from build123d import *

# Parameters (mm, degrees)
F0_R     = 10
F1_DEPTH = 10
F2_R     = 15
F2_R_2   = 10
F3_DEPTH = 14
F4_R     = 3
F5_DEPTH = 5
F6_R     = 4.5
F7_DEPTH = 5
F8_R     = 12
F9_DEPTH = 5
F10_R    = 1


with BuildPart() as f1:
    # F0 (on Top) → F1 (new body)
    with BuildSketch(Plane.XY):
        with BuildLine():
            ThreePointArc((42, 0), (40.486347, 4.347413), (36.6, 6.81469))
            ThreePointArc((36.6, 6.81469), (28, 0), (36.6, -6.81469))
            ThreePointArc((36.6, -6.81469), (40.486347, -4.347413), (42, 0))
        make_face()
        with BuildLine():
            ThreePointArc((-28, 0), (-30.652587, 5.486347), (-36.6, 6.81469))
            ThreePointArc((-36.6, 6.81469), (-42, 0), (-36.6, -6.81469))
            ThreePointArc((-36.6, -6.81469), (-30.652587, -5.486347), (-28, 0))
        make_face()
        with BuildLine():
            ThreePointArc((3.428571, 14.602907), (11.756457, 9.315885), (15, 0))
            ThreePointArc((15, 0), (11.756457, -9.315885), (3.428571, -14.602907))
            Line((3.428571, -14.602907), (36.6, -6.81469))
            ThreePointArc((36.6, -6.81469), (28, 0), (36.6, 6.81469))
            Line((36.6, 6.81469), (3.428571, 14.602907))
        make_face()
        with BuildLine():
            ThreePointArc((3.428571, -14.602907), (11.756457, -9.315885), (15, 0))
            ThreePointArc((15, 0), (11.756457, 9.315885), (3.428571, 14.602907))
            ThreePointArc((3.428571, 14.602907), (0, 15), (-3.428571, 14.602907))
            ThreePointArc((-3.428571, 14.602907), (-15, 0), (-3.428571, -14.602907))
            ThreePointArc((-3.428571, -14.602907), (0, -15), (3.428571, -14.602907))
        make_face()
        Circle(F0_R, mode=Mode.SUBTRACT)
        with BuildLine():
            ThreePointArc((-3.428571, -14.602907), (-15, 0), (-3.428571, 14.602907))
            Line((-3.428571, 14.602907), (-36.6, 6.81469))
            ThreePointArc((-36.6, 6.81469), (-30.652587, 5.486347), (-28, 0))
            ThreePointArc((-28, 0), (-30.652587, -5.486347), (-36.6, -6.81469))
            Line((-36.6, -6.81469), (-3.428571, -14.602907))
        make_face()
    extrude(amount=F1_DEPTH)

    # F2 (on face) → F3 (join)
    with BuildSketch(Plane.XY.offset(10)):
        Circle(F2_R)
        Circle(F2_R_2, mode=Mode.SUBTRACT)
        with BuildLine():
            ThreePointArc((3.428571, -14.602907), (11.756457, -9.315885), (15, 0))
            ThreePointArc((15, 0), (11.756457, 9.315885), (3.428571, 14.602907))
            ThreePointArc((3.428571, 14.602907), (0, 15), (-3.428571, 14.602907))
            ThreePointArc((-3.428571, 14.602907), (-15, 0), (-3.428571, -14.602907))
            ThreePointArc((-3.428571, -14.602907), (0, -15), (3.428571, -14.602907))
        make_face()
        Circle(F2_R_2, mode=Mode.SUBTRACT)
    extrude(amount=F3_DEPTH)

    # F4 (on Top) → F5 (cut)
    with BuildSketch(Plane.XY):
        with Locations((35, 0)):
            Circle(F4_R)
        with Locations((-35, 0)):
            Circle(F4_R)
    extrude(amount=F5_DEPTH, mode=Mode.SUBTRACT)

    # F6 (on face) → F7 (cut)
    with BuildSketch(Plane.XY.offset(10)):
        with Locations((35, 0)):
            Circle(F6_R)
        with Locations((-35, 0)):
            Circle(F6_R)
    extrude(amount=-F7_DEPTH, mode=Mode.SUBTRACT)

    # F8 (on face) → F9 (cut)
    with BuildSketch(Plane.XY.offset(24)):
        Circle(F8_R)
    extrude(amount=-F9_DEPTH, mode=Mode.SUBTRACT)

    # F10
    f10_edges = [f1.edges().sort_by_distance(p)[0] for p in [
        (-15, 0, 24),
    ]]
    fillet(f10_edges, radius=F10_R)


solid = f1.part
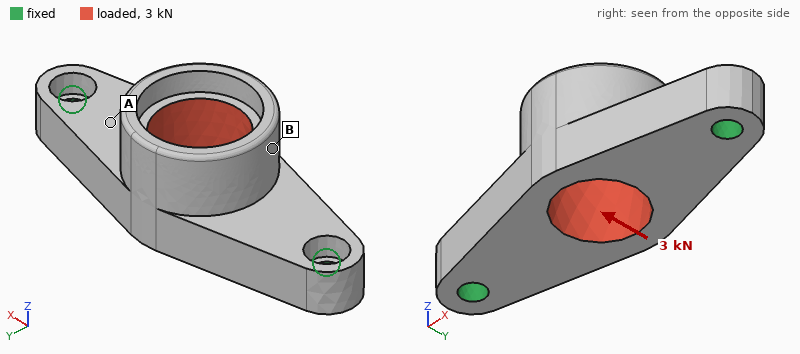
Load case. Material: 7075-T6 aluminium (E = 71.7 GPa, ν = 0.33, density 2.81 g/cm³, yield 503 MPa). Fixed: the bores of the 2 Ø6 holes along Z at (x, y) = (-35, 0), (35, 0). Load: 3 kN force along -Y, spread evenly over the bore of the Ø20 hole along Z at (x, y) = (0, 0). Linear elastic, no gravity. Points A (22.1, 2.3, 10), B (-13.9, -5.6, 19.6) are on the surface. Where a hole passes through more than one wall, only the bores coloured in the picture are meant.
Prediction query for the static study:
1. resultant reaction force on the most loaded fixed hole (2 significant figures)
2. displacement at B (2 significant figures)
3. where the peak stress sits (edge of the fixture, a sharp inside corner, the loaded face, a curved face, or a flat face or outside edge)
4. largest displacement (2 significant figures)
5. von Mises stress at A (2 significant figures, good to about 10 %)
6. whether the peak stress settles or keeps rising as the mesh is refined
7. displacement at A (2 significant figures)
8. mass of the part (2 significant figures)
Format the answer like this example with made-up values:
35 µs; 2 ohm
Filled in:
1.5 kN; 62 µm; edge of the fixture; 82 µm; 41 MPa; keeps rising; 26 µm; 51 g
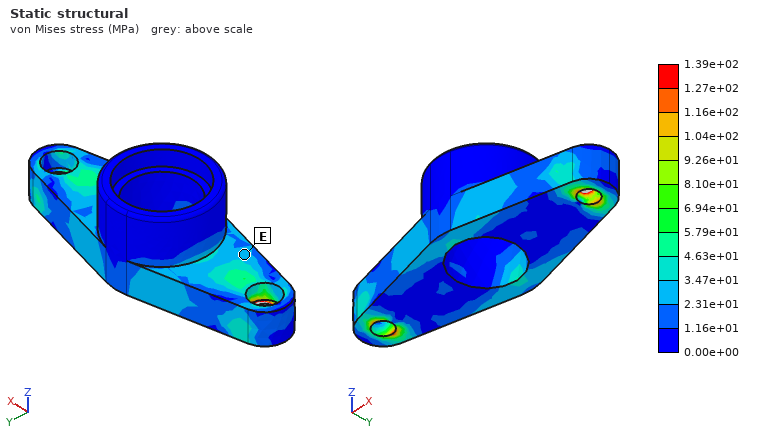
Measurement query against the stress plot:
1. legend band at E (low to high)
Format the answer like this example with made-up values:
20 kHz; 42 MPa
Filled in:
2.31e+01 to 3.47e+01 MPa
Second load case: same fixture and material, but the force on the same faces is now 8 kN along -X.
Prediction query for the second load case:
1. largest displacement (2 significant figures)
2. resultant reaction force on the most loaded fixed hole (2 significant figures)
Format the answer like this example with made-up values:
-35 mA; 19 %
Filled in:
18 µm; 4.1 kN
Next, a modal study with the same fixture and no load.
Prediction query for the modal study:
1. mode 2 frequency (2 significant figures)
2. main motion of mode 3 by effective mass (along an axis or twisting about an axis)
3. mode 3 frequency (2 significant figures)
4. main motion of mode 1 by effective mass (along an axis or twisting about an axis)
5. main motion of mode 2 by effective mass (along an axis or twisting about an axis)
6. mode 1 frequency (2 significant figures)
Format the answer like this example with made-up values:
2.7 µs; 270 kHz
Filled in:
6800 Hz; along Y; 12 kHz; along Y; along Z; 5500 Hz
